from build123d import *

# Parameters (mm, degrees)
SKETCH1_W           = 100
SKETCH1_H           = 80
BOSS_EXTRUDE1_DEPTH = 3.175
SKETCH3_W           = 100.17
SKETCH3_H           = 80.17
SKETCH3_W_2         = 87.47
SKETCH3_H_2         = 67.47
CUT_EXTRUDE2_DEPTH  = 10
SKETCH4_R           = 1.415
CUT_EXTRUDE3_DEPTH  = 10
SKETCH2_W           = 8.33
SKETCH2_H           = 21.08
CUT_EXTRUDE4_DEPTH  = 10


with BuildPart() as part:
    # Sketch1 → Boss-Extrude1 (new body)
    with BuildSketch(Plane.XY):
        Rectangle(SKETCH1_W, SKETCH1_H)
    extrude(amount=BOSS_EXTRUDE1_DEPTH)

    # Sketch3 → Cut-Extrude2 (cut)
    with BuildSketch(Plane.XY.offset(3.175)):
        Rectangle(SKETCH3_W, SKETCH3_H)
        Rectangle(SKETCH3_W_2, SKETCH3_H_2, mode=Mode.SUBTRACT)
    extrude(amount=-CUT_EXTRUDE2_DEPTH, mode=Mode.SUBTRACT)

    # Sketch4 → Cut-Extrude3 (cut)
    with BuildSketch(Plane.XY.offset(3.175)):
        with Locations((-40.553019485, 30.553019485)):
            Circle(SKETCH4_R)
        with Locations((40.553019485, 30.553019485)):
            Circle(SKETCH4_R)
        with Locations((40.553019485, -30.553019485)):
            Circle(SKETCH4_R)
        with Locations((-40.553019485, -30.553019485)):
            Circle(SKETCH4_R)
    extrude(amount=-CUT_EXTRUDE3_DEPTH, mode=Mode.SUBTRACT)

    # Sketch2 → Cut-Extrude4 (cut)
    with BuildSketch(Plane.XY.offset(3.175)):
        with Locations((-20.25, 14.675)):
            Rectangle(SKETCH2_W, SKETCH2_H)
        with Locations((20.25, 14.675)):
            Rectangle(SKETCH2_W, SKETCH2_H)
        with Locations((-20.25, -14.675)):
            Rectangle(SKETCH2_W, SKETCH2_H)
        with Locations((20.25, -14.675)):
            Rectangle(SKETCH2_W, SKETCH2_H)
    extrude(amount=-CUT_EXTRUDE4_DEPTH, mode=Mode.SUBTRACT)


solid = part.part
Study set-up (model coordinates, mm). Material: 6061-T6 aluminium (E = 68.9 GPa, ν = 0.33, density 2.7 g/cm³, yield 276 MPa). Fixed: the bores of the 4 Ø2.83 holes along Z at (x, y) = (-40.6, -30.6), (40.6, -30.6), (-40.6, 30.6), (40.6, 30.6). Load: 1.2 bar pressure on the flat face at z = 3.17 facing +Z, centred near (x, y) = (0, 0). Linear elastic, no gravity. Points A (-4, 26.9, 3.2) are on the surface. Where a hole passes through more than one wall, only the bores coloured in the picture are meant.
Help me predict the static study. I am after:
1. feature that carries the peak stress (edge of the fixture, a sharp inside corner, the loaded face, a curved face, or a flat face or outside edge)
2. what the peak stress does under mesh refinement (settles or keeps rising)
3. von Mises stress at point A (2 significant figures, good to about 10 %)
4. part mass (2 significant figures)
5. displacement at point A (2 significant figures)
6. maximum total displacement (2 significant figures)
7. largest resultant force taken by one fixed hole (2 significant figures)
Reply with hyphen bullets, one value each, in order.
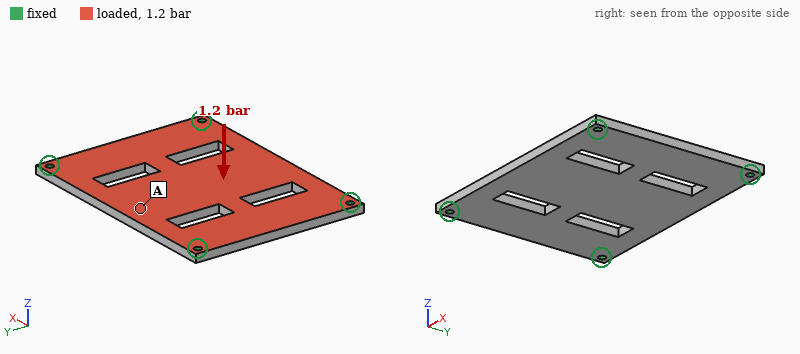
- edge of the fixture
- keeps rising
- 23 MPa
- 44 g
- 0.13 mm
- 0.16 mm
- 160 N
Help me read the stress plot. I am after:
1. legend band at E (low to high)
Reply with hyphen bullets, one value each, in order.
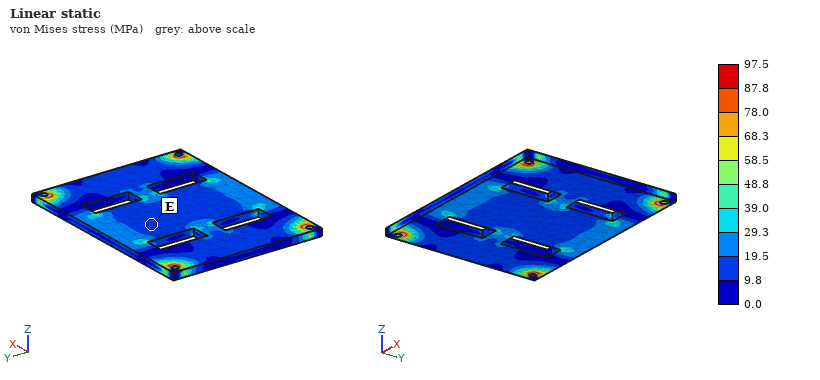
- 9.8 to 19.5 MPa
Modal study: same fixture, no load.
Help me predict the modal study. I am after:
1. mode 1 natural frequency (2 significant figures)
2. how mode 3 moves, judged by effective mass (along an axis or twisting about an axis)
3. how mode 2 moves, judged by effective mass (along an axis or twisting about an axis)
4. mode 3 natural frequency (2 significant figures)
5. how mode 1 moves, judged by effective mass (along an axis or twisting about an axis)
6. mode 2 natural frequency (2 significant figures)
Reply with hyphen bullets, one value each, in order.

- 1700 Hz
- twisting about Y
- twisting about X
- 3800 Hz
- along Z
- 2800 Hz
